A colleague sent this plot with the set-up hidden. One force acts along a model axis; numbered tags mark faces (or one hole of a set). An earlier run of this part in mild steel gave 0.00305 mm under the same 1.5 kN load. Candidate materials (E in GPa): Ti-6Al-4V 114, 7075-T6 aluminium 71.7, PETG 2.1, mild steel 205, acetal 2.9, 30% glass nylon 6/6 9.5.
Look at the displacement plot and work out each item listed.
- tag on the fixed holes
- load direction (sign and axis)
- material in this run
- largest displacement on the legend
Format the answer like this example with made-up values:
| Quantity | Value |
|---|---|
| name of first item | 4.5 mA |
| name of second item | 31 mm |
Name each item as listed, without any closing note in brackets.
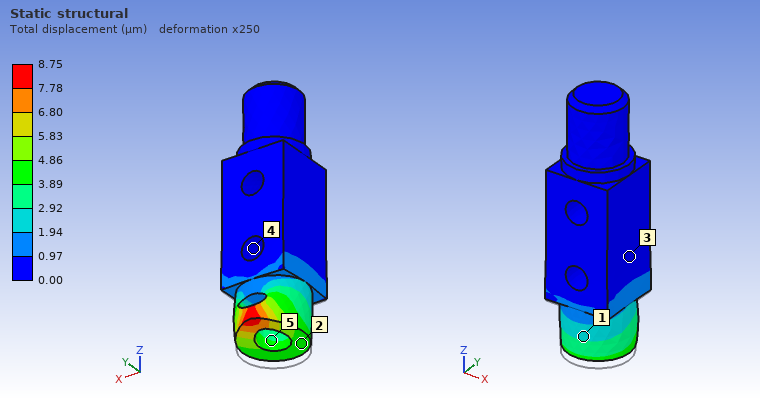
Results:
| Quantity | Value |
|---|---|
| tag on the fixed holes | 4 |
| load direction | +Z |
| material in this run | 7075-T6 aluminium |
| largest displacement on the legend | 8.75 µm |
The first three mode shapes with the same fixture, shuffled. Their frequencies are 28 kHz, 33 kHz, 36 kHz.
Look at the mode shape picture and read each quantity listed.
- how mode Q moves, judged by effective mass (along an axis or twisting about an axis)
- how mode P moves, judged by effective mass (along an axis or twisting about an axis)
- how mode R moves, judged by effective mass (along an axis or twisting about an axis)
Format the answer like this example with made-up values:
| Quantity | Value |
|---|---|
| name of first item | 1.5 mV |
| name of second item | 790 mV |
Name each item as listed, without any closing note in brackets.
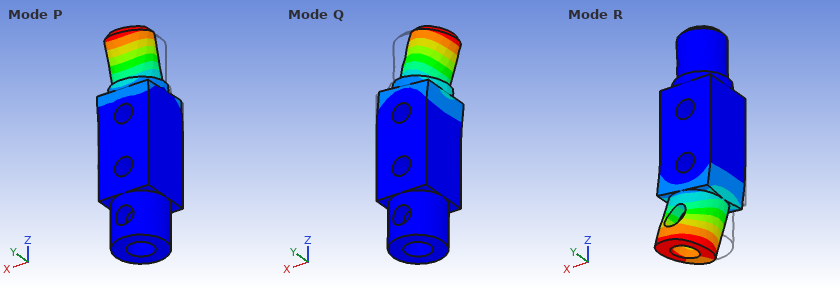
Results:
| Quantity | Value |
|---|---|
| how mode Q moves, judged by effective mass | along X |
| how mode P moves, judged by effective mass | along Y |
| how mode R moves, judged by effective mass | along X |
